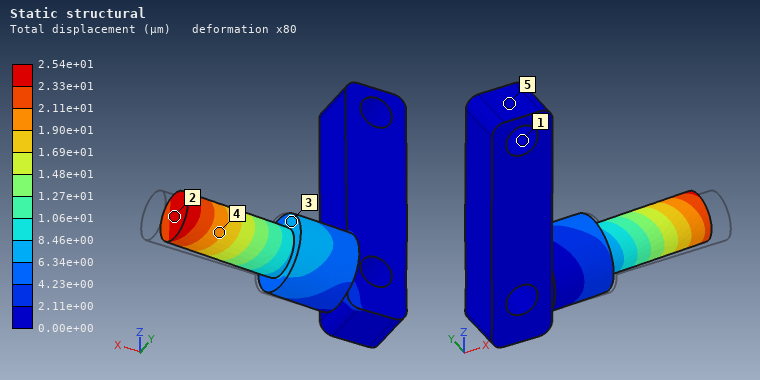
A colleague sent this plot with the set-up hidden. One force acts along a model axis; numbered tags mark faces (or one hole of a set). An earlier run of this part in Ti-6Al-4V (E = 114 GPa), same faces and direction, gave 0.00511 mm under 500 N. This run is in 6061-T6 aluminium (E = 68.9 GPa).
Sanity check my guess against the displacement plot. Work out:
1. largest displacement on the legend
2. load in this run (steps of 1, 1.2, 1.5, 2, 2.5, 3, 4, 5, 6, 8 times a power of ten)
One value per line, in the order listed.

2.54e+01 µm
1.5 kN
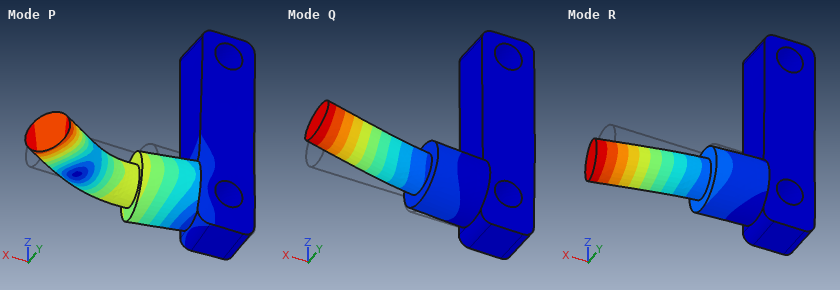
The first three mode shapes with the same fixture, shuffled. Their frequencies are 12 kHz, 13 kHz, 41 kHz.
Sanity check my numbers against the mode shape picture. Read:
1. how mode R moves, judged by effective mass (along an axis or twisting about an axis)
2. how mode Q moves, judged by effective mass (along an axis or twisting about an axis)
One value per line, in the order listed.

along Y
along Z
